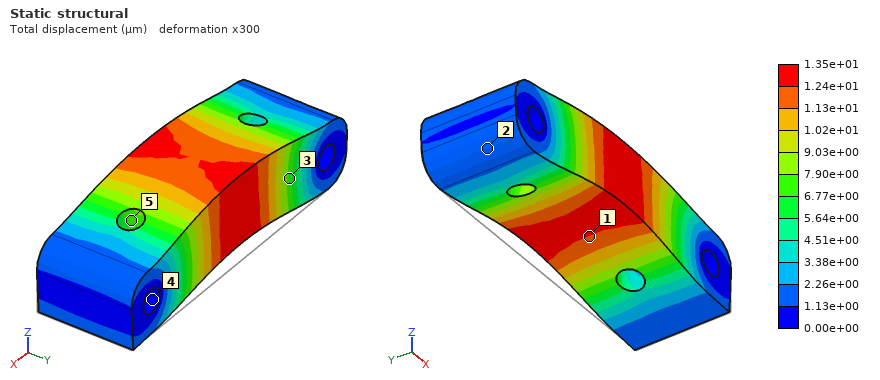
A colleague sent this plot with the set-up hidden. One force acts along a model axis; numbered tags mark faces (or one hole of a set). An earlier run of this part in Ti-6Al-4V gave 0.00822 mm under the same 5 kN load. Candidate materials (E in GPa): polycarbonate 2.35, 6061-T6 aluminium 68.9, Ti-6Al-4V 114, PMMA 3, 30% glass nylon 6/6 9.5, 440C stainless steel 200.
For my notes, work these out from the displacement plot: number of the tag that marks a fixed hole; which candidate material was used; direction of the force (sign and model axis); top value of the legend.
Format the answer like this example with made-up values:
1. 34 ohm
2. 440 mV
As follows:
1. 4
2. 6061-T6 aluminium
3. +Z
4. 1.35e+01 µm
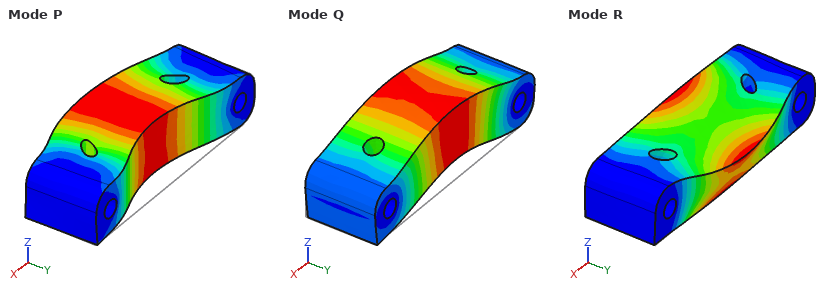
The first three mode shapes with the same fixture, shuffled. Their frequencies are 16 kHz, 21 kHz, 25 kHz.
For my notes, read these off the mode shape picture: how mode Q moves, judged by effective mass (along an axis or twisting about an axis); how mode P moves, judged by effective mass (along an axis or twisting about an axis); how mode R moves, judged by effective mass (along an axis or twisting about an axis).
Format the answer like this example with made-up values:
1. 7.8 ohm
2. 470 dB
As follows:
1. along Z
2. along Y
3. twisting about X
